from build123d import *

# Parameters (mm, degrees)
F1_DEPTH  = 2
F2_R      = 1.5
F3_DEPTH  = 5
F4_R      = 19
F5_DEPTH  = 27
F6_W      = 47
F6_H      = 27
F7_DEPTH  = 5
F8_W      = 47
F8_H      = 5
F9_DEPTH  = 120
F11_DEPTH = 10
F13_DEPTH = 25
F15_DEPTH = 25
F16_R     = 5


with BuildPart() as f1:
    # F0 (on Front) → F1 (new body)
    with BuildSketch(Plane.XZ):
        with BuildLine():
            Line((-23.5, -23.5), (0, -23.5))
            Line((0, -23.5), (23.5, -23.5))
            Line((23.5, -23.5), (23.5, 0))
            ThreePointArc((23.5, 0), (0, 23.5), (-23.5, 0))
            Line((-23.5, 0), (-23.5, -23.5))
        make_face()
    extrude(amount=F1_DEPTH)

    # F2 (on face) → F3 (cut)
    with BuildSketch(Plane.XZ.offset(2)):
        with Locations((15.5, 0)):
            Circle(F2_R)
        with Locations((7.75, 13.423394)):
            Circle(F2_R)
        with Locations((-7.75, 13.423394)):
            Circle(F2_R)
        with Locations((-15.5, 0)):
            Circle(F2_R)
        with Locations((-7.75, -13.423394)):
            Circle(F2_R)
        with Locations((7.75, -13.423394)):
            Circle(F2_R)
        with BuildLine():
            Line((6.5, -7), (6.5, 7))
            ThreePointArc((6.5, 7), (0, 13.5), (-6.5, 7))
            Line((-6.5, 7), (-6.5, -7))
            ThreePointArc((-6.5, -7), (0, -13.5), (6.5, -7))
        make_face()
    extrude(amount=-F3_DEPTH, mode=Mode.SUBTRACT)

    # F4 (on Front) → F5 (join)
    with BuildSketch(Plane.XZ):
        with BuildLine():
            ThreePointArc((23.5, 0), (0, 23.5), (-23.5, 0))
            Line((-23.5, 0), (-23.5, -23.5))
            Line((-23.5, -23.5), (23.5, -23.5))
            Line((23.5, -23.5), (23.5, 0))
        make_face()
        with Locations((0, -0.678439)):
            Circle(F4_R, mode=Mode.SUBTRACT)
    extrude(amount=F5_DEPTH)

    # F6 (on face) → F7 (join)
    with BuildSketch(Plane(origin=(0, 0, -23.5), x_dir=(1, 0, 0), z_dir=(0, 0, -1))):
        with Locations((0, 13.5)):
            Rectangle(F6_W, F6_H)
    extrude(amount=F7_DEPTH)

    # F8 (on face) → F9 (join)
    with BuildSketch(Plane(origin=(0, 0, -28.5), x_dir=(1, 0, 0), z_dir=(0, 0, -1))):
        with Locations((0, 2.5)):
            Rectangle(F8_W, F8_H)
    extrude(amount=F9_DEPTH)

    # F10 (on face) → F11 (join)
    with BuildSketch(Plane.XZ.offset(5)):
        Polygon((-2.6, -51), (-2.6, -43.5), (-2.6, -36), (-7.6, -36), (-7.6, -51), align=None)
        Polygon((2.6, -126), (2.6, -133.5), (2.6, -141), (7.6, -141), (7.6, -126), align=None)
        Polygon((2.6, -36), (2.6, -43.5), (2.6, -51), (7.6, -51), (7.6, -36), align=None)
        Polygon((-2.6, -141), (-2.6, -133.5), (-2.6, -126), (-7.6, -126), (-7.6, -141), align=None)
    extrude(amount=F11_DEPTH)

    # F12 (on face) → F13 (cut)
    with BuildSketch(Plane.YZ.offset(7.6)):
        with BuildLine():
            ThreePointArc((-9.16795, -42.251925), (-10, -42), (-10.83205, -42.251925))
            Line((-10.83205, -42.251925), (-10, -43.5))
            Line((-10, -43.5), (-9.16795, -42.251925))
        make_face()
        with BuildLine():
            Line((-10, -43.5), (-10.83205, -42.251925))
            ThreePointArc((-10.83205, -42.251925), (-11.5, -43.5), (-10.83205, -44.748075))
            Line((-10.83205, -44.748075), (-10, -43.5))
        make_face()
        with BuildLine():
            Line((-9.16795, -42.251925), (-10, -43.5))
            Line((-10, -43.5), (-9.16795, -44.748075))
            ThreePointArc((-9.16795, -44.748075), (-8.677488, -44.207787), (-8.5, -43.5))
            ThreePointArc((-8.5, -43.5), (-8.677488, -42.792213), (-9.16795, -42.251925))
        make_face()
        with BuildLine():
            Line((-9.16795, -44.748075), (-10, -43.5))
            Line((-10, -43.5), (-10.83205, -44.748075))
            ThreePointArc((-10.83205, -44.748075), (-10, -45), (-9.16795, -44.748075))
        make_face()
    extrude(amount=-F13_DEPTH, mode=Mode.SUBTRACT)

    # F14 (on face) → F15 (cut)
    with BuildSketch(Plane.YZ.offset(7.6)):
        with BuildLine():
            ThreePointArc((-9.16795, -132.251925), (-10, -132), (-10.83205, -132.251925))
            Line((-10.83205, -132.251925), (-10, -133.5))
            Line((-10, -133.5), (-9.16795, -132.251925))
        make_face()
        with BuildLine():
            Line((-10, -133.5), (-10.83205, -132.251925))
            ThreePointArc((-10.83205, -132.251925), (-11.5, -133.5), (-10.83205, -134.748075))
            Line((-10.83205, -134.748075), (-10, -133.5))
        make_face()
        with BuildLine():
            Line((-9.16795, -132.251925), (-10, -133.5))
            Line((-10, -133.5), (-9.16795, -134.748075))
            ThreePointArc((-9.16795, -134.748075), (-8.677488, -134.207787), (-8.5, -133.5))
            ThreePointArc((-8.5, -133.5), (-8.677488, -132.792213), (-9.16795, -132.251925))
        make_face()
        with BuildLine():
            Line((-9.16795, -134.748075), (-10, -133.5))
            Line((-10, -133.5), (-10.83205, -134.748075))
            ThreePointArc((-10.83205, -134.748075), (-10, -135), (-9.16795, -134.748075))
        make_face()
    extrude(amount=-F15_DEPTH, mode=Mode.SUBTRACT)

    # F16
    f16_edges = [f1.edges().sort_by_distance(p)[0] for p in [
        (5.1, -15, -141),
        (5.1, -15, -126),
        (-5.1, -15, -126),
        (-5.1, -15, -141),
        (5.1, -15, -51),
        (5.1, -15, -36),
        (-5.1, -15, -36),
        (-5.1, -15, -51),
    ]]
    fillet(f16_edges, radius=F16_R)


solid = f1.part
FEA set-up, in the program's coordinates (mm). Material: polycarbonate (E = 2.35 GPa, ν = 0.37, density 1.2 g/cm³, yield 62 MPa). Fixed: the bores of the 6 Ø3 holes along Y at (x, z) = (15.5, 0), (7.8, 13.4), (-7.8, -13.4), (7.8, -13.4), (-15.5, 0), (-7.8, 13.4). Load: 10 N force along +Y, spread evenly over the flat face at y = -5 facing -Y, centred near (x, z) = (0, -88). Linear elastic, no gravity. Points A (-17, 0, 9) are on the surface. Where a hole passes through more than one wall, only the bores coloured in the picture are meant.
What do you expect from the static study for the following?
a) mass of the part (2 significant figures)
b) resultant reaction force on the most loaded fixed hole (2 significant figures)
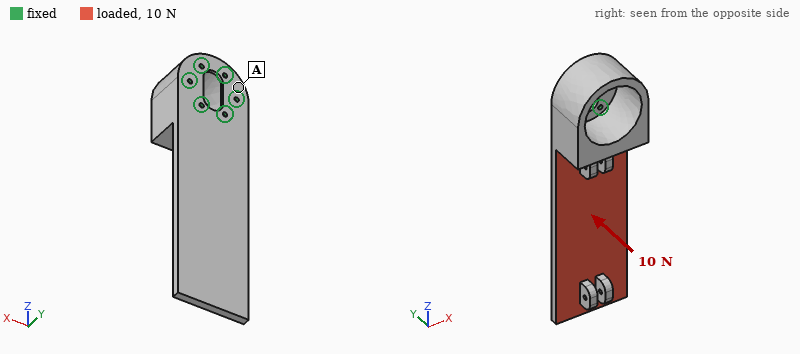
74 g
18 N
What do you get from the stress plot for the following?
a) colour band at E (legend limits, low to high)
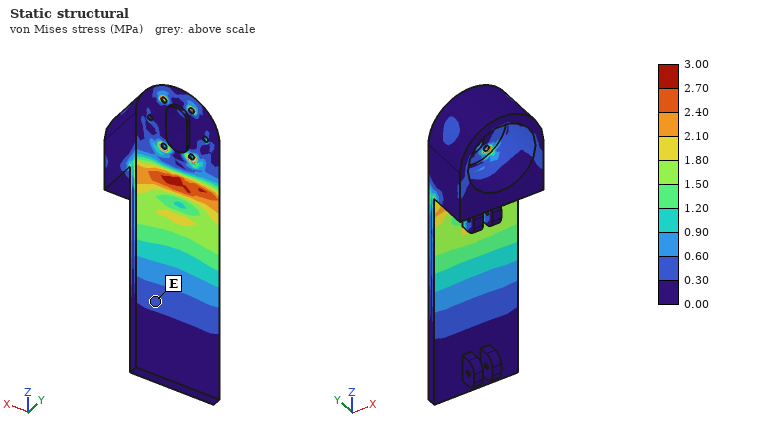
0.30 to 0.60 MPa
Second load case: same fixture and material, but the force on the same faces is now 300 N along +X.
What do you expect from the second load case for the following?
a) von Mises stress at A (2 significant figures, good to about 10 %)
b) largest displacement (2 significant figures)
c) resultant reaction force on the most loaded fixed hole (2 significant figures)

5.9 MPa
1.8 mm
380 N
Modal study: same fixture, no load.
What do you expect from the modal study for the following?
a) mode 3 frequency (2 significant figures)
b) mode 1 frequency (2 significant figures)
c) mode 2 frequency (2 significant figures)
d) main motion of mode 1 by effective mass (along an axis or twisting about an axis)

430 Hz
73 Hz
380 Hz
along Y
